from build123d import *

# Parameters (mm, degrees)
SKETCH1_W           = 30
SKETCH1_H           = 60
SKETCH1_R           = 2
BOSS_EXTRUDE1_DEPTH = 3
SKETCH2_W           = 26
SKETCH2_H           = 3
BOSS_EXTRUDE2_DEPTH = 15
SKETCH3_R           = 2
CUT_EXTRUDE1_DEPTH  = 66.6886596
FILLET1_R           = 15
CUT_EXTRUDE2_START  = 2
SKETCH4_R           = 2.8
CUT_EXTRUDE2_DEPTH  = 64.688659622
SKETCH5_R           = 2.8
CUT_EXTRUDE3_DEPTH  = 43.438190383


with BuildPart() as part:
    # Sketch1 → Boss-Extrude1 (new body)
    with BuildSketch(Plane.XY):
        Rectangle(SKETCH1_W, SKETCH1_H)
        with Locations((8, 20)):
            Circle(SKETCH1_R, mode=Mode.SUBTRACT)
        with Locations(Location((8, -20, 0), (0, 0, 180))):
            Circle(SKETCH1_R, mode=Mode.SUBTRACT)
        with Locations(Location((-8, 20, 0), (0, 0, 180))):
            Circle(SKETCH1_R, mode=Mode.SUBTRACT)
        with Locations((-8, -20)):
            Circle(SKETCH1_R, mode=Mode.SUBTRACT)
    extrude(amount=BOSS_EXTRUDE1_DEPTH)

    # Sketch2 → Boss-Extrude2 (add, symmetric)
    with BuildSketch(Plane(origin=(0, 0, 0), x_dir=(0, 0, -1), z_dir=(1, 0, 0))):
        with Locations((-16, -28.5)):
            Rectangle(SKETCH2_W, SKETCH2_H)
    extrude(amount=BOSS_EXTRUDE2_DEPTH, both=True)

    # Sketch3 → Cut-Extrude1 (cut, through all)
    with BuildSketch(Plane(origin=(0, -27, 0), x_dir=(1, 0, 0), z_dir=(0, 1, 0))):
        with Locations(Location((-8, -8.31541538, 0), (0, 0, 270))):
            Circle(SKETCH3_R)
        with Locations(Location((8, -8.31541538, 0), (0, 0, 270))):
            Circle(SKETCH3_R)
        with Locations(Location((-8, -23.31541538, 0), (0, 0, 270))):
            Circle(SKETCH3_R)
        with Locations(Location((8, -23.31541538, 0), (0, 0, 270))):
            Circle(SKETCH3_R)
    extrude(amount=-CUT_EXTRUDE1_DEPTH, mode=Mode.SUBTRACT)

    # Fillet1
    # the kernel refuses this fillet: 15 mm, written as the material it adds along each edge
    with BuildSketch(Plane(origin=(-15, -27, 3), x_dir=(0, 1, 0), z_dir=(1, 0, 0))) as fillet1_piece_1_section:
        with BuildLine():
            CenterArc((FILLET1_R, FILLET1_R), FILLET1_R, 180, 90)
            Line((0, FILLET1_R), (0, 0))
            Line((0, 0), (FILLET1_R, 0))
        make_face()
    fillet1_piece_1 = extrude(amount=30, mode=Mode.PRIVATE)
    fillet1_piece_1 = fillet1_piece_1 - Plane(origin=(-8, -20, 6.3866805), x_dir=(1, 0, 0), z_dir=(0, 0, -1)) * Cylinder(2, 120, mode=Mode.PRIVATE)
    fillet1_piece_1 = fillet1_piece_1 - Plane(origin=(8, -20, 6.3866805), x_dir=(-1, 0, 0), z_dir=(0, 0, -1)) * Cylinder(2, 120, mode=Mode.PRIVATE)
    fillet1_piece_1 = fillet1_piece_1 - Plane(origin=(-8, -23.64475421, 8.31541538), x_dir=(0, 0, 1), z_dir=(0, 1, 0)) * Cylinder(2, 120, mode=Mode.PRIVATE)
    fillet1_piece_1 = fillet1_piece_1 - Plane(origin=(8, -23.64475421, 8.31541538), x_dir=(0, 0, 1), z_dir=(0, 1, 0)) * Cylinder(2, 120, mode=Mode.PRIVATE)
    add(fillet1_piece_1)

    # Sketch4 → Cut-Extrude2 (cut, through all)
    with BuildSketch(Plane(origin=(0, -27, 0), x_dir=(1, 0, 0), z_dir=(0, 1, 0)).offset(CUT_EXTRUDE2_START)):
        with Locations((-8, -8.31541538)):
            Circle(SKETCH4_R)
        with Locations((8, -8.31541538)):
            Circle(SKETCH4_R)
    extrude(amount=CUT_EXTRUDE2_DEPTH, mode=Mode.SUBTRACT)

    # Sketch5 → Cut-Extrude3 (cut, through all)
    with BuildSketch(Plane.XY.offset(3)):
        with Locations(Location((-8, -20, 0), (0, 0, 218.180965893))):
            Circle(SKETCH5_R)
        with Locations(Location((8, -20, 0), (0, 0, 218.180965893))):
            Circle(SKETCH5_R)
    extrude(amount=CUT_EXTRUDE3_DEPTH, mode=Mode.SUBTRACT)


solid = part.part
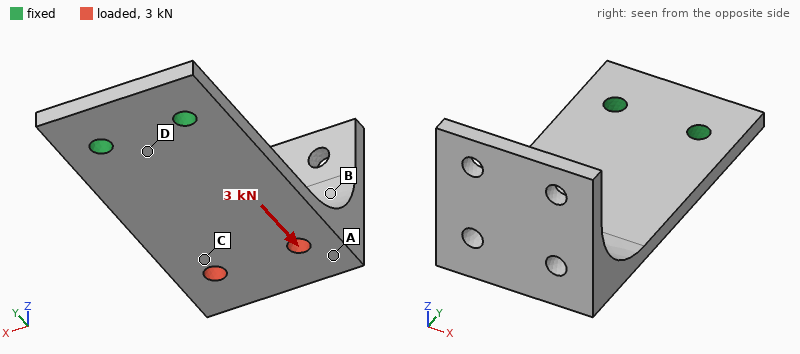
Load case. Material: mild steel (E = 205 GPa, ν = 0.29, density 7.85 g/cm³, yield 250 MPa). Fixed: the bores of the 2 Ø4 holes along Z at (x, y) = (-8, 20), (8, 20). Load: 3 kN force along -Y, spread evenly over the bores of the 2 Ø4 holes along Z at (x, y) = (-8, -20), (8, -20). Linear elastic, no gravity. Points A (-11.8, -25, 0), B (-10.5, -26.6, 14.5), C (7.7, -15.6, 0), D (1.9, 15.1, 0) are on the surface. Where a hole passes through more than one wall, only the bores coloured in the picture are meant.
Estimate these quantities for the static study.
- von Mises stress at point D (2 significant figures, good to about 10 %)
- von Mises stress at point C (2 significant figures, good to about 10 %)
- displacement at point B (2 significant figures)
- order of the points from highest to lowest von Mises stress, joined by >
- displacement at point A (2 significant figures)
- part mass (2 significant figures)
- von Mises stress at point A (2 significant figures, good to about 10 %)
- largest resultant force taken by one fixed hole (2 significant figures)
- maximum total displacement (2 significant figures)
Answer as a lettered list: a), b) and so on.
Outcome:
a) 24 MPa
b) 45 MPa
c) 4.0 µm
d) C > D > A > B
e) 7.4 µm
f) 68 g
g) 13 MPa
h) 1.5 kN
i) 8.0 µm
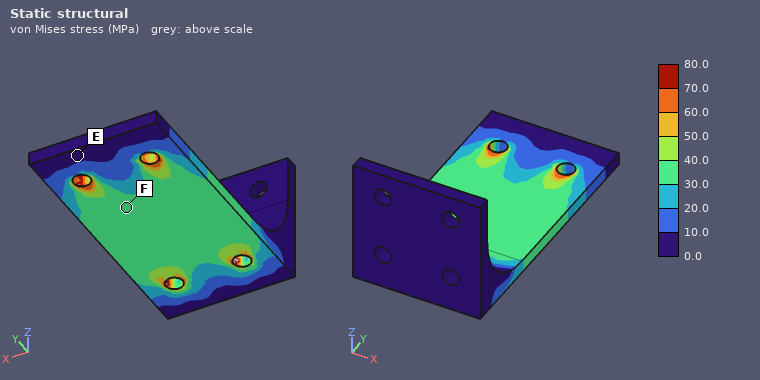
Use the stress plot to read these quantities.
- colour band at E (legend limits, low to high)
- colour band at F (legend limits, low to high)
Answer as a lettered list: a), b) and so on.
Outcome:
a) 0.0 to 10.0 MPa
b) 30.0 to 40.0 MPa
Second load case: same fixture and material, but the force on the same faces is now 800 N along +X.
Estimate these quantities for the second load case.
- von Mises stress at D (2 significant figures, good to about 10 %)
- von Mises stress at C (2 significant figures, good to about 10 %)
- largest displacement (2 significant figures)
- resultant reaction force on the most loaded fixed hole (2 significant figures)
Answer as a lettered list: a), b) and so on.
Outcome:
a) 27 MPa
b) 21 MPa
c) 27 µm
d) 1.8 kN
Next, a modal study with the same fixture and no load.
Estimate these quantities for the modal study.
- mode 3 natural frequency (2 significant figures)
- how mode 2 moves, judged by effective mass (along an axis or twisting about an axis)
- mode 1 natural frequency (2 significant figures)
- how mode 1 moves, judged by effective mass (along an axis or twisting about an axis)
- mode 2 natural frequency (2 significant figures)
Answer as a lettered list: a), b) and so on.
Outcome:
a) 3000 Hz
b) along X
c) 520 Hz
d) along Z
e) 1500 Hz
